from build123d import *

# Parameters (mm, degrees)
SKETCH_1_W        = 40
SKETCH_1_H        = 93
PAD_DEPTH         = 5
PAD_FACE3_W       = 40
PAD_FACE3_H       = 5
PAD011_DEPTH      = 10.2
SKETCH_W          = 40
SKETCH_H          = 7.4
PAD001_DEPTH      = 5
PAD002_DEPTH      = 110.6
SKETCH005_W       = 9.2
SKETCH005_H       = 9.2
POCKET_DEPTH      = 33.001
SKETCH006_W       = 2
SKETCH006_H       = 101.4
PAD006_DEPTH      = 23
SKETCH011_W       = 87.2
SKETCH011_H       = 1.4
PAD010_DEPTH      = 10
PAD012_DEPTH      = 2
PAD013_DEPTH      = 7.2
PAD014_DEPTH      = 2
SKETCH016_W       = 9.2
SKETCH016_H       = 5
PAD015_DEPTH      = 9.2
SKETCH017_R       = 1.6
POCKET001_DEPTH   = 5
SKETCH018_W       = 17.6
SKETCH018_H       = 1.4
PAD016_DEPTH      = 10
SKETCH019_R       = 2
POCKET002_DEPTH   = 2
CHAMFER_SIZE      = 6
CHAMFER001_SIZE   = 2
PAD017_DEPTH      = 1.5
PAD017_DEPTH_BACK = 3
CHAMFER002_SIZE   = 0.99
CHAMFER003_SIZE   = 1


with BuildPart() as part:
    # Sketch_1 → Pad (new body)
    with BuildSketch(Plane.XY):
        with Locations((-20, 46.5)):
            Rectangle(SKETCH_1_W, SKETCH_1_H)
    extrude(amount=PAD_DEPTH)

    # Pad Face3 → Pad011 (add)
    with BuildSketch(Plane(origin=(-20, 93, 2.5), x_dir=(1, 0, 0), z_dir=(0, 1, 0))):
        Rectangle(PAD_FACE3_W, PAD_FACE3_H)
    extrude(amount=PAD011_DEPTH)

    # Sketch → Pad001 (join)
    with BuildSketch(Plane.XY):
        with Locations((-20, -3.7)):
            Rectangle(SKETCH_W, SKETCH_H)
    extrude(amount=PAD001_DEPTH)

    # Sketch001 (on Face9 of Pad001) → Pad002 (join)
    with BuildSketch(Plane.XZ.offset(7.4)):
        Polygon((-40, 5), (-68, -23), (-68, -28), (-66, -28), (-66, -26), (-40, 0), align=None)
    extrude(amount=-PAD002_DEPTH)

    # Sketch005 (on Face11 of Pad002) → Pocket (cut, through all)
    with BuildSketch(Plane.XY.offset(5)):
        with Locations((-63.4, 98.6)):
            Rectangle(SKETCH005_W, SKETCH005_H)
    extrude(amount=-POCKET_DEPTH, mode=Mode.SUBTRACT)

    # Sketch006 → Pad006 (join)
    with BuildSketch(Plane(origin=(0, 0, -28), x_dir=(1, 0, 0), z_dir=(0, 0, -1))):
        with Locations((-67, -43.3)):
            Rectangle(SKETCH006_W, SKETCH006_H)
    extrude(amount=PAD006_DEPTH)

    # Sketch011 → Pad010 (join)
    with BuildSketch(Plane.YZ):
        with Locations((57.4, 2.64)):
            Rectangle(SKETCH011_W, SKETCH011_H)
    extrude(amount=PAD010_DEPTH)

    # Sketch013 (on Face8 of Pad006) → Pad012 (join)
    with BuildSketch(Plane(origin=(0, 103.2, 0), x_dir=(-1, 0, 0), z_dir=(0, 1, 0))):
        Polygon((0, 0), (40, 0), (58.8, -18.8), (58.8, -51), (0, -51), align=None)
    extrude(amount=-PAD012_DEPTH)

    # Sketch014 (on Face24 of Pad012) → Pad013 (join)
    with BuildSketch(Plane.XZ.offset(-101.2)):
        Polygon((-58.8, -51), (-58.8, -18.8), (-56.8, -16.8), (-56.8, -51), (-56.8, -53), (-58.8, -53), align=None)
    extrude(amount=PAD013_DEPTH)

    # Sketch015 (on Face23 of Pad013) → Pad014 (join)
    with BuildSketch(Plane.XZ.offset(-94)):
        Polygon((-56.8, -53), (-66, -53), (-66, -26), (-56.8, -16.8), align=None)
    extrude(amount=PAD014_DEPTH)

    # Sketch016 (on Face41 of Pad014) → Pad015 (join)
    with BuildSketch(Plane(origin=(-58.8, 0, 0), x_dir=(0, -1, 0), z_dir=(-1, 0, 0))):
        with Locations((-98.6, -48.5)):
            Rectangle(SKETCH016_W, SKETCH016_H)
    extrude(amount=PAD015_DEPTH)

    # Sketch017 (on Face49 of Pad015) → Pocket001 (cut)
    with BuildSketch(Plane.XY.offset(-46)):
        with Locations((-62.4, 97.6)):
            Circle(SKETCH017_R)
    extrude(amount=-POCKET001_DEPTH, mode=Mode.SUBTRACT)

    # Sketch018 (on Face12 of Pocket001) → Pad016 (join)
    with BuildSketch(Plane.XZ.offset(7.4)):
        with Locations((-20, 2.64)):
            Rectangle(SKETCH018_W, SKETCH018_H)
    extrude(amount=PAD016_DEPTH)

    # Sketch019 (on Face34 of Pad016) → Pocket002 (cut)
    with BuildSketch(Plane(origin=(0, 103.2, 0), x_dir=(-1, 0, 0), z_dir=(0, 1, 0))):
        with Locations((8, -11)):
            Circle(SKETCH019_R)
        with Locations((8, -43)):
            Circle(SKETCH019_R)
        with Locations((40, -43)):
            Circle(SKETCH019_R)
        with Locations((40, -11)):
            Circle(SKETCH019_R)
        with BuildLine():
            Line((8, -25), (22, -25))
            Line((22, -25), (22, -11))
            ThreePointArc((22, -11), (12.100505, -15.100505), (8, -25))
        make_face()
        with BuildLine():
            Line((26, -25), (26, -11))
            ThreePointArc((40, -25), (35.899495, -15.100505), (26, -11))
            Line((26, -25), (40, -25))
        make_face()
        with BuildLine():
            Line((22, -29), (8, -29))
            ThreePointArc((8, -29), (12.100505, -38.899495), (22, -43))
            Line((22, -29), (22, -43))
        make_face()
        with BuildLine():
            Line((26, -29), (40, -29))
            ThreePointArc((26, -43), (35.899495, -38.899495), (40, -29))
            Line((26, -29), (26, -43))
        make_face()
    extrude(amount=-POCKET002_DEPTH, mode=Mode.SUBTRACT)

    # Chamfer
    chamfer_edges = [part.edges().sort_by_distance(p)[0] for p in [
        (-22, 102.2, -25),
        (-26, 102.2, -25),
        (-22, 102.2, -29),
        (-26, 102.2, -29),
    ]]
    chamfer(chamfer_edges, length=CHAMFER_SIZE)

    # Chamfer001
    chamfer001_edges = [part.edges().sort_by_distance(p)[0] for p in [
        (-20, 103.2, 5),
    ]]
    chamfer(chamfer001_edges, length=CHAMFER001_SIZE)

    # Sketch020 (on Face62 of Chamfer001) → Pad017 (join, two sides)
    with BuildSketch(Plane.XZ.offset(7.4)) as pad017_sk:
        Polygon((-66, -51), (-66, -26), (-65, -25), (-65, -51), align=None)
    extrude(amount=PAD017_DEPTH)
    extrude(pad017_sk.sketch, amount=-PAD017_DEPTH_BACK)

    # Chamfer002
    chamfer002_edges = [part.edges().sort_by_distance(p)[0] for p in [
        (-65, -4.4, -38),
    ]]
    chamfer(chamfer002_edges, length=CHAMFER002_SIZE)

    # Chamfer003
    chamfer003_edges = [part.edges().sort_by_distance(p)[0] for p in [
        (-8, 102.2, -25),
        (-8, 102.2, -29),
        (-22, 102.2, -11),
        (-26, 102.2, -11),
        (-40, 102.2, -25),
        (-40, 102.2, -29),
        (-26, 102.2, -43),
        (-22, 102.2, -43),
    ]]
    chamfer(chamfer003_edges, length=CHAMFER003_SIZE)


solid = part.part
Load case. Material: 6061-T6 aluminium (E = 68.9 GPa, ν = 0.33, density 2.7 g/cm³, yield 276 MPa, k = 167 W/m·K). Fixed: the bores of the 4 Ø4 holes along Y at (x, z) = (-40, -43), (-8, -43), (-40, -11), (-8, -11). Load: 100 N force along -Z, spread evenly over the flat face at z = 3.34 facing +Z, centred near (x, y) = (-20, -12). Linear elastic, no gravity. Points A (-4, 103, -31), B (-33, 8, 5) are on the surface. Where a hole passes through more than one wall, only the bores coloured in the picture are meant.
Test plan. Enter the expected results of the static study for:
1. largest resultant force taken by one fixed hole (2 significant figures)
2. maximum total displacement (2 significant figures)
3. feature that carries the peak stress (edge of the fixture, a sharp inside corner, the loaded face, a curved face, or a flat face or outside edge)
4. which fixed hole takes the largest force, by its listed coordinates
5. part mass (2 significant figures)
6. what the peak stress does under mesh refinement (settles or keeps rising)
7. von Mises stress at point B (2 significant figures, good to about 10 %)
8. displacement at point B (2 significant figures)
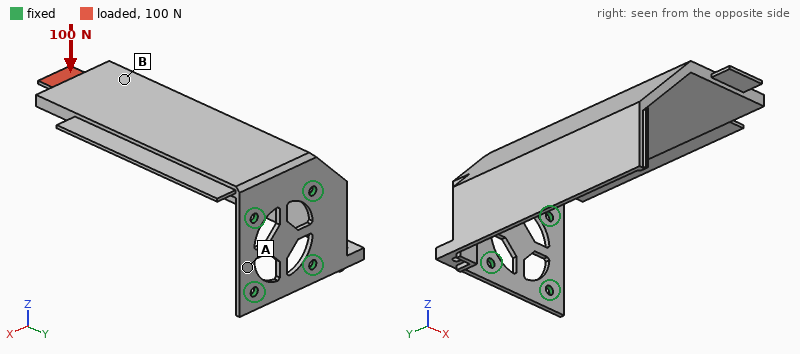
330 N
1.6 mm
edge of the fixture
(-40, -11)
130 g
keeps rising
19 MPa
1.1 mm
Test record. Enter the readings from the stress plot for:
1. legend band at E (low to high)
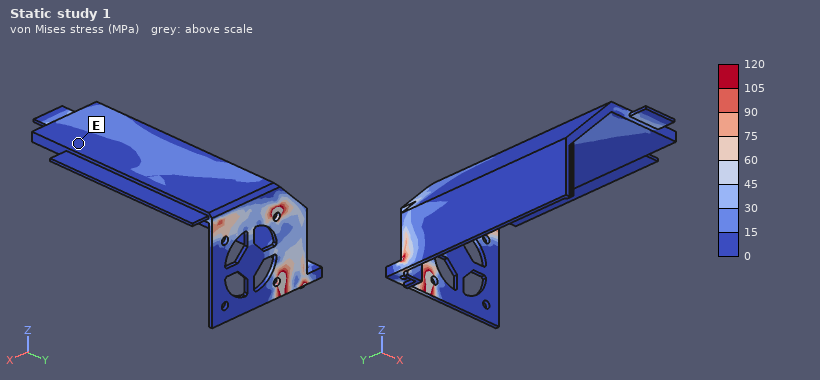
0 to 15 MPa
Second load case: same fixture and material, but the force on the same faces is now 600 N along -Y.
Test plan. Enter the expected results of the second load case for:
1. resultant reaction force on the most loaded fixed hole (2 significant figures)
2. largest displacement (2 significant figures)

390 N
0.73 mm
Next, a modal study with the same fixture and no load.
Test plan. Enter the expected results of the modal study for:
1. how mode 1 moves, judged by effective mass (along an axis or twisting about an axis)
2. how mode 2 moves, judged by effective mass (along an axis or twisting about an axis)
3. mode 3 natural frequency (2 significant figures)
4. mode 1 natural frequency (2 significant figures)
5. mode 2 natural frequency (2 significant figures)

along Z
along X
840 Hz
240 Hz
410 Hz
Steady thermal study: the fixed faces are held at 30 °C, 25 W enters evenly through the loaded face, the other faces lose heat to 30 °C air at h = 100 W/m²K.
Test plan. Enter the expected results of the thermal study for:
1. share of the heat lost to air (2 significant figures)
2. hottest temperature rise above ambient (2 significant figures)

86 %
64 K
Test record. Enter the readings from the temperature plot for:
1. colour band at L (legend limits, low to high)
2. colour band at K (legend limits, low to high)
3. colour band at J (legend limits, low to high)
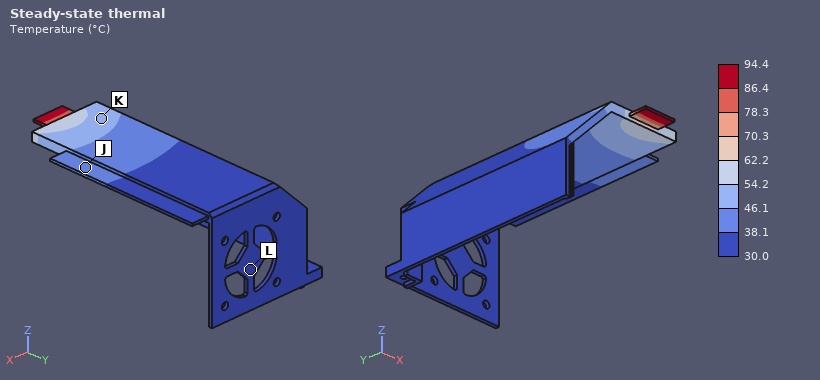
30.0 to 38.1 °C
46.1 to 54.2 °C
38.1 to 46.1 °C
